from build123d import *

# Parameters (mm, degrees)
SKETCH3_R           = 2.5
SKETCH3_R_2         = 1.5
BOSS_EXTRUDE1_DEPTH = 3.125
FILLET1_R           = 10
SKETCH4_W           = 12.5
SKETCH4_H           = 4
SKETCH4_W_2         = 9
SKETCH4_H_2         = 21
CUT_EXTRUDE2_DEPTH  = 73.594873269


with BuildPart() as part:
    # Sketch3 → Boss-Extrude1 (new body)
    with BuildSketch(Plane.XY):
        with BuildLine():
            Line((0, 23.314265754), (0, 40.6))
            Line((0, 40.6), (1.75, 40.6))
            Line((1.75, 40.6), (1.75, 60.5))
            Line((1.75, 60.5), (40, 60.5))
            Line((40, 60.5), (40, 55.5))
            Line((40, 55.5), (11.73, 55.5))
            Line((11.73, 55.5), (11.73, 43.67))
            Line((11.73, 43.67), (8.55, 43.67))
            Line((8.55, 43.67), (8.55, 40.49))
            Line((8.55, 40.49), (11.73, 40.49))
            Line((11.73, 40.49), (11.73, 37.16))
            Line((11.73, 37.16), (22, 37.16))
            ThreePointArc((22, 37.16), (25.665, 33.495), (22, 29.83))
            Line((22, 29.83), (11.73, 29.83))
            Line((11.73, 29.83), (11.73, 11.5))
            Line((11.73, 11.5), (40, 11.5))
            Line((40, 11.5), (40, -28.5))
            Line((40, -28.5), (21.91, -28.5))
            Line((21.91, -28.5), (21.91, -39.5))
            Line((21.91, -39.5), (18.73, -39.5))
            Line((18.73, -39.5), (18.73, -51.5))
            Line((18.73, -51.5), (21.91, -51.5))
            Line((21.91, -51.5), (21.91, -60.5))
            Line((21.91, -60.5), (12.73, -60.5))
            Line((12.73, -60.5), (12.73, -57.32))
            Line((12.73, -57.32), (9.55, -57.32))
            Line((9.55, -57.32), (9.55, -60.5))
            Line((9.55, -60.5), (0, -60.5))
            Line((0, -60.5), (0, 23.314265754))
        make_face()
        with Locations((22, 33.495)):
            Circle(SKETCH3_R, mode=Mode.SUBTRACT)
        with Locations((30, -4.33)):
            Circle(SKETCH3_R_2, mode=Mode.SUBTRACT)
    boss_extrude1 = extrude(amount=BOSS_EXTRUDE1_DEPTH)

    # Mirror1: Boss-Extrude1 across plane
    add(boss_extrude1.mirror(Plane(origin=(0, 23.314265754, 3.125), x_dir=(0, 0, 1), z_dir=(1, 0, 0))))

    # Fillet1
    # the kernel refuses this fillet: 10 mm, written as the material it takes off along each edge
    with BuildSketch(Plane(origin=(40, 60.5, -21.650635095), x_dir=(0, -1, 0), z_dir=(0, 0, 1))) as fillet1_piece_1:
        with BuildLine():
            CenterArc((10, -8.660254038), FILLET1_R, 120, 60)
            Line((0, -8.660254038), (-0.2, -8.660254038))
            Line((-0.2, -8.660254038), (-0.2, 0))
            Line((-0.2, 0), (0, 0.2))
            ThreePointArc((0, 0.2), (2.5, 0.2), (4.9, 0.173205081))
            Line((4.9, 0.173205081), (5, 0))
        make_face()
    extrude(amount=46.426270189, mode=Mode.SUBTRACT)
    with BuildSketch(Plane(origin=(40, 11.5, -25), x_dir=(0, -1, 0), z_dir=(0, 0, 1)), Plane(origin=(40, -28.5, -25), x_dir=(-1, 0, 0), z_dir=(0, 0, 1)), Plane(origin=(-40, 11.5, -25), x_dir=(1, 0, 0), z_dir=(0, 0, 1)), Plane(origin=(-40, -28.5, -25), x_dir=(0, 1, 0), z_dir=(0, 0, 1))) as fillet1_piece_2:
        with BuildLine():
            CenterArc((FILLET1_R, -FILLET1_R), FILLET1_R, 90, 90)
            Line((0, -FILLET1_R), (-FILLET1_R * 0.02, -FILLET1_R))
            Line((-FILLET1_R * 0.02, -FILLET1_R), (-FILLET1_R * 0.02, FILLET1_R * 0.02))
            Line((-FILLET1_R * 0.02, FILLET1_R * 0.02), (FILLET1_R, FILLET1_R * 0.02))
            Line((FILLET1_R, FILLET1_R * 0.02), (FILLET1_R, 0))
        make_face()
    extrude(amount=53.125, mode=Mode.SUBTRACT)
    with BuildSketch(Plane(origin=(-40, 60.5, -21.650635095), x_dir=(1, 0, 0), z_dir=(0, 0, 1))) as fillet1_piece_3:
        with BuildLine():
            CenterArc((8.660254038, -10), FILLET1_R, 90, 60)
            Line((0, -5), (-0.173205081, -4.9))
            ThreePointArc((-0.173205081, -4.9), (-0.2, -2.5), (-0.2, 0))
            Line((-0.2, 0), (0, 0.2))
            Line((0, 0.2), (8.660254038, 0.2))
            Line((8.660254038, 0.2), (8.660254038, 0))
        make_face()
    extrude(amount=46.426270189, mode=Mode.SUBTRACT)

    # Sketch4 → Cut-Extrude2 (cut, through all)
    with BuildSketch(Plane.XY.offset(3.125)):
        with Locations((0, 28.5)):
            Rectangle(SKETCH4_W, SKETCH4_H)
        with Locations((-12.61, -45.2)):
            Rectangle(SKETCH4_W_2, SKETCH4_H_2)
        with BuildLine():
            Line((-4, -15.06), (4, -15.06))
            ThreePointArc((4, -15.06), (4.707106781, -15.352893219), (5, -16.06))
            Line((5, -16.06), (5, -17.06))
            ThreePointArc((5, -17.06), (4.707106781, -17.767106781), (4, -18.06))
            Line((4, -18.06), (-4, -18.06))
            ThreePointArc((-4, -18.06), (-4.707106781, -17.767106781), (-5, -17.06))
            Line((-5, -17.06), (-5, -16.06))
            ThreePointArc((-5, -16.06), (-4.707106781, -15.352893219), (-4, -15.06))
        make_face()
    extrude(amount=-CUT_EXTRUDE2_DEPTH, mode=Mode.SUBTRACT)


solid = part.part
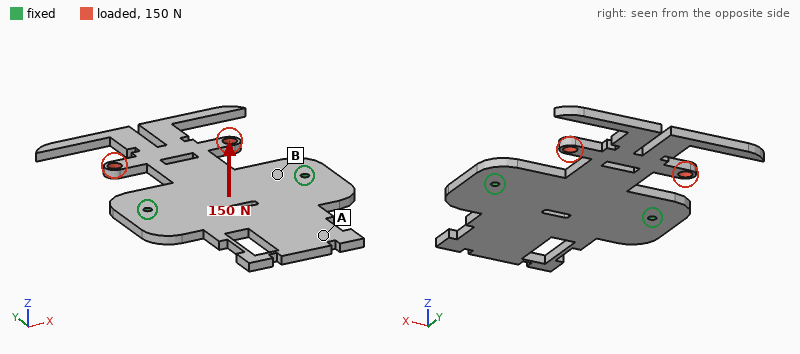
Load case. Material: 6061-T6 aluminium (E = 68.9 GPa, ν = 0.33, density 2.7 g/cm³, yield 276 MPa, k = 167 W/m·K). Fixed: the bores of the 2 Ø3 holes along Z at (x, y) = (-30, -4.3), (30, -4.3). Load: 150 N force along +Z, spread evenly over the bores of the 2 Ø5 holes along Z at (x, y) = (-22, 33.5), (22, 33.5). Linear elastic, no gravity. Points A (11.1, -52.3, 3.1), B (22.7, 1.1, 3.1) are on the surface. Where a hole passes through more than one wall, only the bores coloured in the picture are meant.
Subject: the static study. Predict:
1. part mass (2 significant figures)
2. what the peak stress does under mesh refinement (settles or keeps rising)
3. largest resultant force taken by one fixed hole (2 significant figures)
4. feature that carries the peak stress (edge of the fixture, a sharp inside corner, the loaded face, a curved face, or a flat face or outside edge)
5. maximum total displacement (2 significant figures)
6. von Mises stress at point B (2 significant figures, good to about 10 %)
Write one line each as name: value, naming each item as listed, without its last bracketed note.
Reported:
part mass: 47 g
what the peak stress does under mesh refinement: keeps rising
largest resultant force taken by one fixed hole: 75 N
feature that carries the peak stress: edge of the fixture
maximum total displacement: 1.3 mm
von Mises stress at point B: 48 MPa
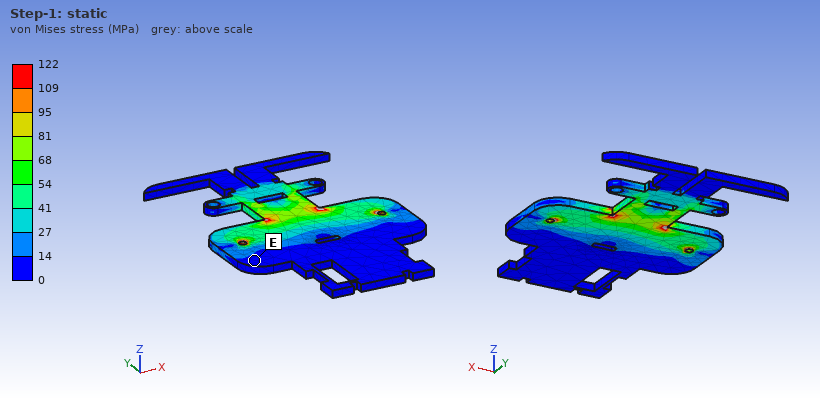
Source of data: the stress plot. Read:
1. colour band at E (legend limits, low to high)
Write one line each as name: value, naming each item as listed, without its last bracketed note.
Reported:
colour band at E: 0 to 14 MPa
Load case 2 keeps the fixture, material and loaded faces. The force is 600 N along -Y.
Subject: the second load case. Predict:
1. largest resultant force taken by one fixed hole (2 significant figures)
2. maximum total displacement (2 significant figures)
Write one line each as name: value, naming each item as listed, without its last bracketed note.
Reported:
largest resultant force taken by one fixed hole: 300 N
maximum total displacement: 78 µm
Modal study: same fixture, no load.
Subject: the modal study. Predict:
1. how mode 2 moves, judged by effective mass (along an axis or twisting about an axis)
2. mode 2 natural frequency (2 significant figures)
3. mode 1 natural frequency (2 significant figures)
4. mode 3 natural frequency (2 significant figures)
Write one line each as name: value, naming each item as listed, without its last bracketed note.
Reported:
how mode 2 moves, judged by effective mass: along Z
mode 2 natural frequency: 900 Hz
mode 1 natural frequency: 470 Hz
mode 3 natural frequency: 1000 Hz
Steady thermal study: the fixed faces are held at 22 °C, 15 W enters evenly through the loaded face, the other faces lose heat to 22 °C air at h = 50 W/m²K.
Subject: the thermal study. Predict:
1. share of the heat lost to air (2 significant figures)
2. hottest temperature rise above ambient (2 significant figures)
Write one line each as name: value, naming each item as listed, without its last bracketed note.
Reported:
share of the heat lost to air: 50 %
hottest temperature rise above ambient: 67 K
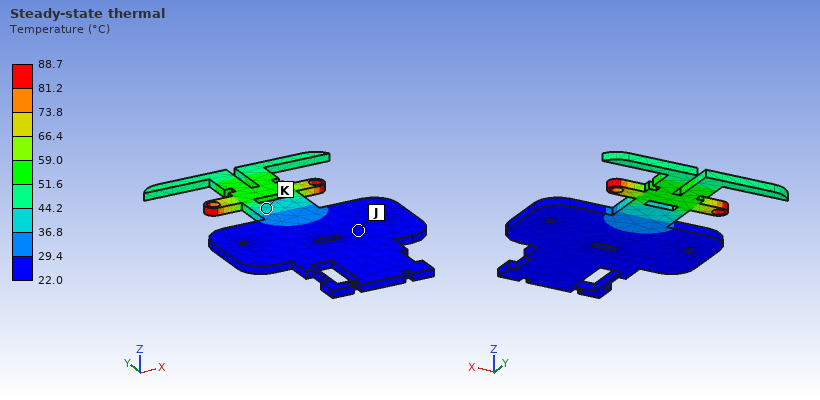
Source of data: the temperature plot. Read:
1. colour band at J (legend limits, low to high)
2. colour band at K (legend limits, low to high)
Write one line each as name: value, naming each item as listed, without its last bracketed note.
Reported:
colour band at J: 22.0 to 29.4 °C
colour band at K: 36.8 to 44.2 °C
